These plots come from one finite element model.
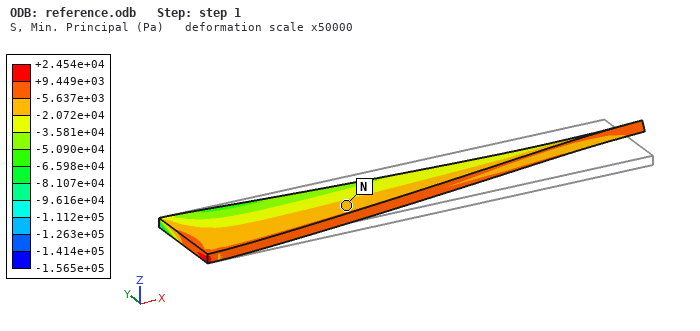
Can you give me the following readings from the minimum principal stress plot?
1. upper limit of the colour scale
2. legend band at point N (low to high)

+2.454e+04 Pa
-2.072e+04 to -5.637e+03 Pa
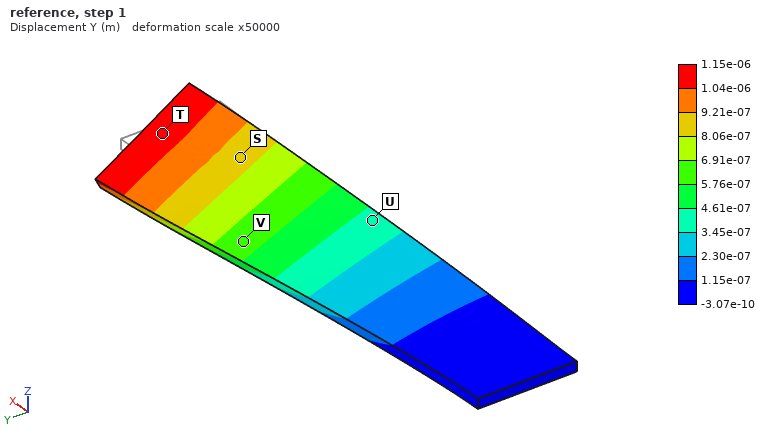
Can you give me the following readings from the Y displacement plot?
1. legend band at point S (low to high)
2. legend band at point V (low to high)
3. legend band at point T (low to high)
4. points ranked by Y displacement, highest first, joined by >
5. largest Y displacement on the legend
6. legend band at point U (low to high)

8.06e-07 to 9.21e-07 m
5.76e-07 to 6.91e-07 m
1.04e-06 to 1.15e-06 m
T > S > V > U
1.15e-06 m
3.45e-07 to 4.61e-07 m
